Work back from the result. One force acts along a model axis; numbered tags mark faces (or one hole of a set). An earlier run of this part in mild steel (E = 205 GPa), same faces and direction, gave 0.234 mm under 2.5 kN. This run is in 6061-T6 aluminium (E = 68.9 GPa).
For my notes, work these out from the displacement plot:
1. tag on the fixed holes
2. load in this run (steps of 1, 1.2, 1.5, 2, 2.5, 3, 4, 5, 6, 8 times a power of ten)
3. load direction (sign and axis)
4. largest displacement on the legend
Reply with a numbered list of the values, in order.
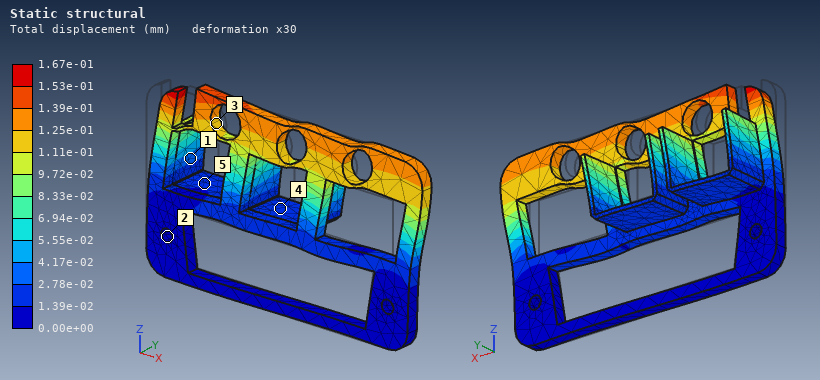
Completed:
1. 2
2. 600 N
3. +X
4. 1.67e-01 mm
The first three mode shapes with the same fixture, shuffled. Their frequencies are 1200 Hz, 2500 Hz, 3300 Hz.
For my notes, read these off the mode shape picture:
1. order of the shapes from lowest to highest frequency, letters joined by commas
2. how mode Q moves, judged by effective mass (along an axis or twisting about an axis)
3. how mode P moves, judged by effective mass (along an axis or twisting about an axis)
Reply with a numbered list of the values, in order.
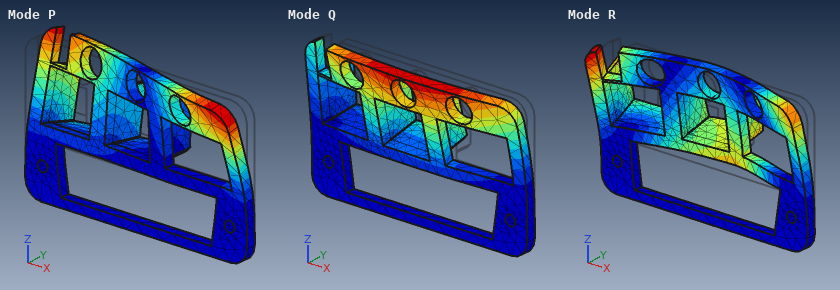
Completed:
1. Q, P, R
2. along Y
3. twisting about Z
